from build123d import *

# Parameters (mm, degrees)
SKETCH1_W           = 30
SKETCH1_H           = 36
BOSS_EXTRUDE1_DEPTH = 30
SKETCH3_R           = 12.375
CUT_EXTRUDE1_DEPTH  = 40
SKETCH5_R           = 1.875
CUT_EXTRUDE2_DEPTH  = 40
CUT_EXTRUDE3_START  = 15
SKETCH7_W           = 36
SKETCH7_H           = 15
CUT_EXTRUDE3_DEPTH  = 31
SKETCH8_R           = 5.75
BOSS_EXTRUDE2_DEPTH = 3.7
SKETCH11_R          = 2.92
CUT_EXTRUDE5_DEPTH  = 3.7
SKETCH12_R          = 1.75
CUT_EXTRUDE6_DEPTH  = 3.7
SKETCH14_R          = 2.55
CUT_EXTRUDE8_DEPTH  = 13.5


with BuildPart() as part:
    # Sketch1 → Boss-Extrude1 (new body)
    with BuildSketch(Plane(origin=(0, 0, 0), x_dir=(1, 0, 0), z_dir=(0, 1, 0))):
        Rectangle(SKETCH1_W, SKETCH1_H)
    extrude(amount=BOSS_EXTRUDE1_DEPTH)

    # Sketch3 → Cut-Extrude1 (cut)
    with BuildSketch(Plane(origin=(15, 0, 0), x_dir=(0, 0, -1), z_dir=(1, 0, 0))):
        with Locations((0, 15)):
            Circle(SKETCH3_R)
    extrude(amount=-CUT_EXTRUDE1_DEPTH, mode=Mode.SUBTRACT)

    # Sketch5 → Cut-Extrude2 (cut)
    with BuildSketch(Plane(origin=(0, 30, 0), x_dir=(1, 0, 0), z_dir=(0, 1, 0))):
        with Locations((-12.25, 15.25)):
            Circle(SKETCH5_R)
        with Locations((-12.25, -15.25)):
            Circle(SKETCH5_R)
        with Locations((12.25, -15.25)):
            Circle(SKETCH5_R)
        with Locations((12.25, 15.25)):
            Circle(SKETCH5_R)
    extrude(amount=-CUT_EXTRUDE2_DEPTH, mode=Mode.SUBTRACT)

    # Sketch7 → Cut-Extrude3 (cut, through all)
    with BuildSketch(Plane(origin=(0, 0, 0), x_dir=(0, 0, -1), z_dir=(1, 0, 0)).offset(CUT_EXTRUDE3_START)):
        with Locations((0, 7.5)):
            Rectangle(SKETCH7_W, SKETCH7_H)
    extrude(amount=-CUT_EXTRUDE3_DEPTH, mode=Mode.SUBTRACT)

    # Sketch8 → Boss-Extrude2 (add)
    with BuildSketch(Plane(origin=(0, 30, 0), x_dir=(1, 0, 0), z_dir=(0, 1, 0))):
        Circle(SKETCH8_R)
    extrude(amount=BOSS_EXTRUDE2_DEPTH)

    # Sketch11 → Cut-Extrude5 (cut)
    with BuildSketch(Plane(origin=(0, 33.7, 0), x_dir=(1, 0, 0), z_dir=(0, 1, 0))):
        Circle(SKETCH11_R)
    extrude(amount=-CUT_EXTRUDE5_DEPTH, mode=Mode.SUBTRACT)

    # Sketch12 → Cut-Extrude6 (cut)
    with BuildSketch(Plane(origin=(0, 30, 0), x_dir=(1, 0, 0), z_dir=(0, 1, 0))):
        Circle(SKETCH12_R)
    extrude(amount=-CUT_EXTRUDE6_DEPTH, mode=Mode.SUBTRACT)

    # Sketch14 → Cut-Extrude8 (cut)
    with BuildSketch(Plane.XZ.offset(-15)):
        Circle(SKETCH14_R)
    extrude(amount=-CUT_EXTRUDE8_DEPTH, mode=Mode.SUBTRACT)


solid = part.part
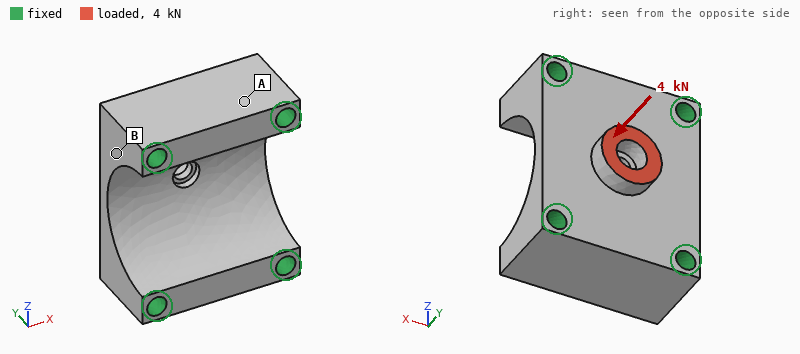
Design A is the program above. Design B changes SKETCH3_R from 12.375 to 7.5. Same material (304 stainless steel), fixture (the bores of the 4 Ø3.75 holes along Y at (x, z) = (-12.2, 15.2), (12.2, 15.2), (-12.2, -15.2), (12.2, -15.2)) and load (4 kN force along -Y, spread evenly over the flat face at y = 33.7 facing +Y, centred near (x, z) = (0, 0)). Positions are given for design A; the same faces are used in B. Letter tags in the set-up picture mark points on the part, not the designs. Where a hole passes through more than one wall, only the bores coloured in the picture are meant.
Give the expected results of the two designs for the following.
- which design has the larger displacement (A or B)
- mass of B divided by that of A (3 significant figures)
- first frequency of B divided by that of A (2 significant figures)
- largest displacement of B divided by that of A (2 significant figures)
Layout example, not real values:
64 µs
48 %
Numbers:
A
1.52
1.0
0.44
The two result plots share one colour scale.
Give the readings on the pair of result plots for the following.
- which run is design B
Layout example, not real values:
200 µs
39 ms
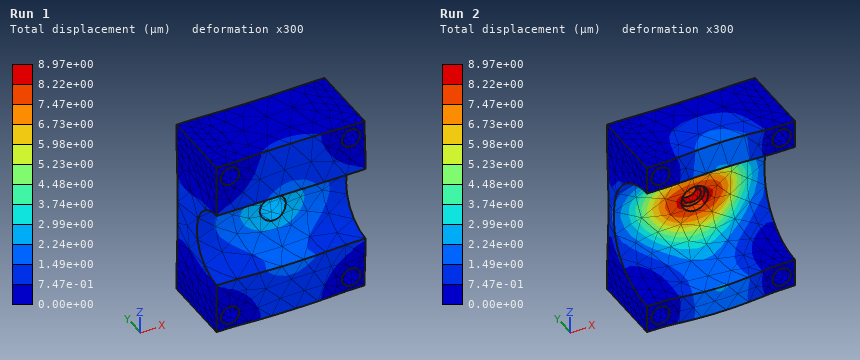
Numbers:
Run 1
